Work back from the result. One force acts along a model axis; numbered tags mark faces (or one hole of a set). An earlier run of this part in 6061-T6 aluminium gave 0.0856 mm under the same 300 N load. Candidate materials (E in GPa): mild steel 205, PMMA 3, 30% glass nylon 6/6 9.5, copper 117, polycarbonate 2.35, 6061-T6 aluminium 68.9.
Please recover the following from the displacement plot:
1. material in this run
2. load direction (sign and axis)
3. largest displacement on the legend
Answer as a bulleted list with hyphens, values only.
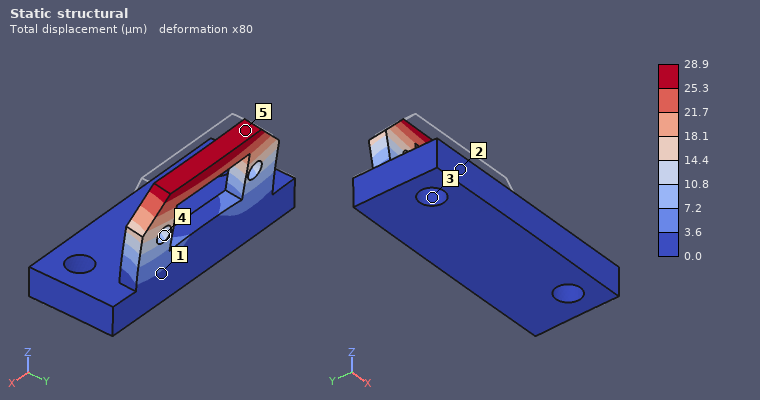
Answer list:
- mild steel
- +Y
- 28.9 µm
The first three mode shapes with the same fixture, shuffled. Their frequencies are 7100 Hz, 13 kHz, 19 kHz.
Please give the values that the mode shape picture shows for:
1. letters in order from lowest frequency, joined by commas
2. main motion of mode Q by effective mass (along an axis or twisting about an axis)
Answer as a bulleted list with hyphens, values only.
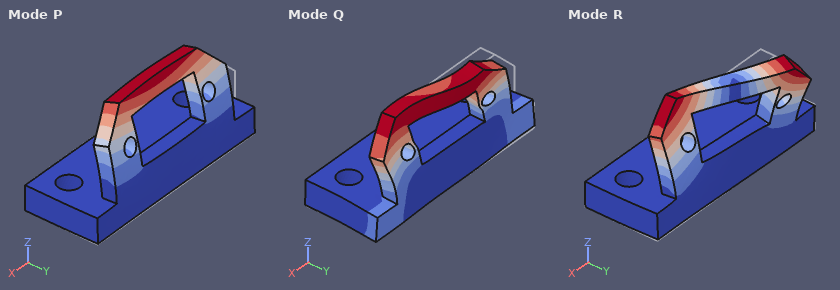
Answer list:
- P, R, Q
- along X
